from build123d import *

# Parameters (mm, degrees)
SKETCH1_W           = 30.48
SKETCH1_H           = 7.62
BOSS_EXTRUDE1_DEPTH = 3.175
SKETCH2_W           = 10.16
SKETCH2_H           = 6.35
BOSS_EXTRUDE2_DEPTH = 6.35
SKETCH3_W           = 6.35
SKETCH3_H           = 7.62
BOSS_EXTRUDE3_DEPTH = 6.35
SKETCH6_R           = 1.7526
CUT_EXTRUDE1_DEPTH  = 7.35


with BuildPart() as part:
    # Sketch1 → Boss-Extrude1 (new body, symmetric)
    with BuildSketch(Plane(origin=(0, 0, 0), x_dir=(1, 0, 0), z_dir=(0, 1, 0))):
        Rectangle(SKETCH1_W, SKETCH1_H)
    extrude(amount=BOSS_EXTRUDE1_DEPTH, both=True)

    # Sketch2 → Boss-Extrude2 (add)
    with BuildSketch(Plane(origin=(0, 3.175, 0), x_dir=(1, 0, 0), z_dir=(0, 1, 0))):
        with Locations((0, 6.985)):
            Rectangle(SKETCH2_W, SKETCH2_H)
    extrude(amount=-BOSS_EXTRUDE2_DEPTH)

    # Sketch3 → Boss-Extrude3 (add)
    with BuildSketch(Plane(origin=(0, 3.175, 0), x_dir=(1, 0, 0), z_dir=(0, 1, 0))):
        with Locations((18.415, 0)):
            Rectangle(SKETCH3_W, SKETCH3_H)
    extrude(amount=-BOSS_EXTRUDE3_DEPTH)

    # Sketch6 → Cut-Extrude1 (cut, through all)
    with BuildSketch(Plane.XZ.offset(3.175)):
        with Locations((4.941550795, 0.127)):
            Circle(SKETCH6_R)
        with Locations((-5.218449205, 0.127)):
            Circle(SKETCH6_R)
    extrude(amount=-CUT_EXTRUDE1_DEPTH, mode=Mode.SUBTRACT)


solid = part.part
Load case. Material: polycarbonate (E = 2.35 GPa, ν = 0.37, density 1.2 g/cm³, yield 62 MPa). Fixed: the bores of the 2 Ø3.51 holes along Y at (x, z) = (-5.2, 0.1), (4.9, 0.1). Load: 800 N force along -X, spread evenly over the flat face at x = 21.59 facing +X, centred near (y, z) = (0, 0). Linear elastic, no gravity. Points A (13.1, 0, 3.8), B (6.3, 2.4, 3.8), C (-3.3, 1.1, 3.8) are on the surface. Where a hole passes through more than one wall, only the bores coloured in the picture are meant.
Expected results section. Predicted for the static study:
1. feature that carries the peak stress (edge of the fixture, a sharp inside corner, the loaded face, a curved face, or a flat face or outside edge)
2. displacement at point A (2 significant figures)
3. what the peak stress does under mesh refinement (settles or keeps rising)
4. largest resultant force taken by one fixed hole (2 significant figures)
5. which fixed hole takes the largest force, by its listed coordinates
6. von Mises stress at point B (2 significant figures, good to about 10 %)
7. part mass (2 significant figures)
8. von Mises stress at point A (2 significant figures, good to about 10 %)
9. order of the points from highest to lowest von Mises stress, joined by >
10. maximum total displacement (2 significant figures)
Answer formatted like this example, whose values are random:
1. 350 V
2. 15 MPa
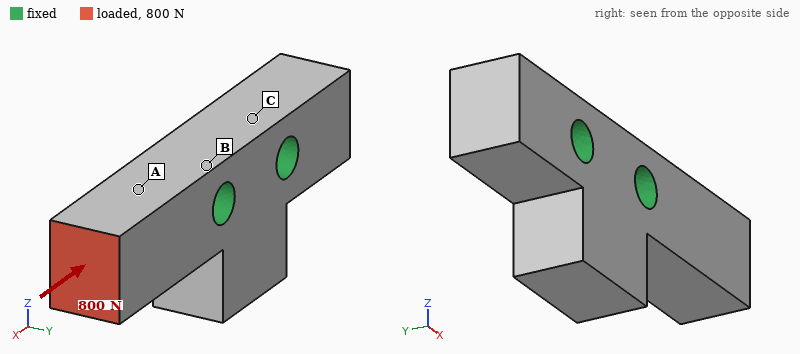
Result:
1. edge of the fixture
2. 0.052 mm
3. keeps rising
4. 760 N
5. (4.9, 0.1)
6. 8.6 MPa
7. 2.5 g
8. 16 MPa
9. A > B > C
10. 0.11 mm
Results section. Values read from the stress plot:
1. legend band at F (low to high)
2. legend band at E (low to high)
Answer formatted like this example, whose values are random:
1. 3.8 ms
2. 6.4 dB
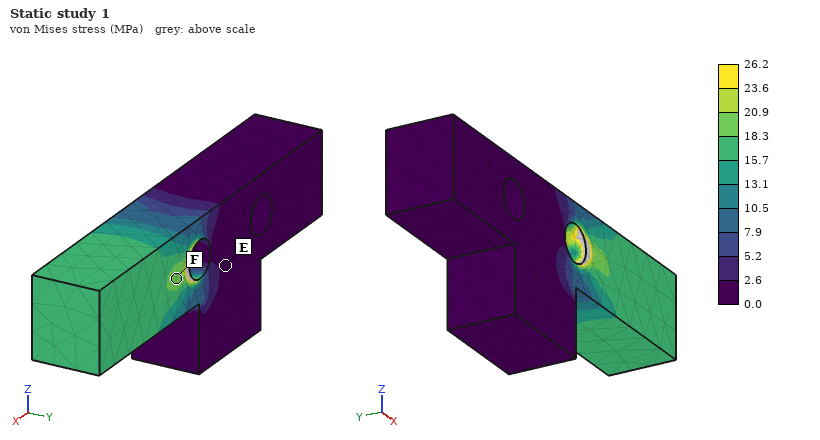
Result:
1. 18.3 to 20.9 MPa
2. 0.0 to 2.6 MPa
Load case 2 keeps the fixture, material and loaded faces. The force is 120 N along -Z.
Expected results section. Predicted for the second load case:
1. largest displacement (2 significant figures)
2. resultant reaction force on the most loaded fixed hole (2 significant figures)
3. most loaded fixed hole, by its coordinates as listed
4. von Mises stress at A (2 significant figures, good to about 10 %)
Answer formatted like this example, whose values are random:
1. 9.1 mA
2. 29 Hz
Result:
1. 0.44 mm
2. 180 N
3. (4.9, 0.1)
4. 17 MPa
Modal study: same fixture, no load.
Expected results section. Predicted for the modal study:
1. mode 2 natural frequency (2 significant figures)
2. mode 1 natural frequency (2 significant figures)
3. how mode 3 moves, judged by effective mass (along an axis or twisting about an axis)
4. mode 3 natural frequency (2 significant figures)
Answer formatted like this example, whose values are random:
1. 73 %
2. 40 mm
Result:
1. 5200 Hz
2. 5200 Hz
3. twisting about X
4. 12 kHz
